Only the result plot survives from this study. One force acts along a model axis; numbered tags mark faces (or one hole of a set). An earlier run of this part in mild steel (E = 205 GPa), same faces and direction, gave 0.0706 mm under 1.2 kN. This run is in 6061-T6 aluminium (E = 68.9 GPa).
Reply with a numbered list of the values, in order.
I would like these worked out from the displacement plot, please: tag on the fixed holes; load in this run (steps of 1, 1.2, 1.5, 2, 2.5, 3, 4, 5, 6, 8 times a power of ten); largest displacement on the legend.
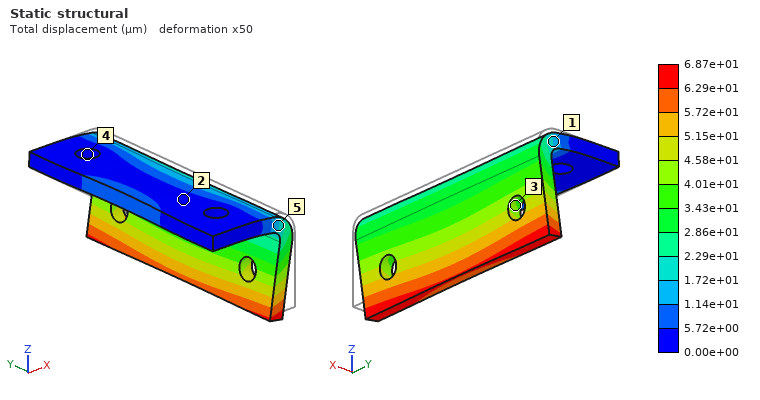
1. 4
2. 400 N
3. 6.87e+01 µm
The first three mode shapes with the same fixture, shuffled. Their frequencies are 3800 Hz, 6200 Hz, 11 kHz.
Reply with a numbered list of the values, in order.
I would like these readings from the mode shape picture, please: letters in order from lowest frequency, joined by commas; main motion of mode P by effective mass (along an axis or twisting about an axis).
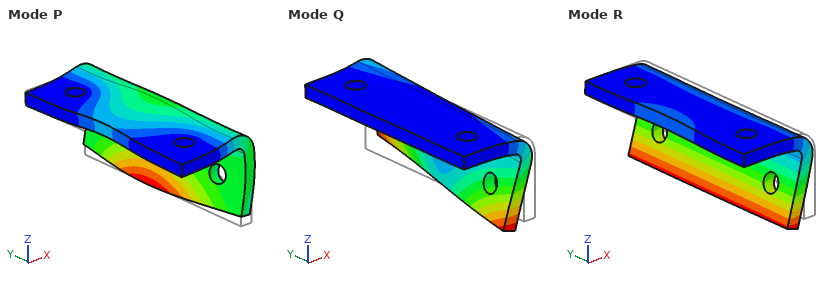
1. R, Q, P
2. along Z
